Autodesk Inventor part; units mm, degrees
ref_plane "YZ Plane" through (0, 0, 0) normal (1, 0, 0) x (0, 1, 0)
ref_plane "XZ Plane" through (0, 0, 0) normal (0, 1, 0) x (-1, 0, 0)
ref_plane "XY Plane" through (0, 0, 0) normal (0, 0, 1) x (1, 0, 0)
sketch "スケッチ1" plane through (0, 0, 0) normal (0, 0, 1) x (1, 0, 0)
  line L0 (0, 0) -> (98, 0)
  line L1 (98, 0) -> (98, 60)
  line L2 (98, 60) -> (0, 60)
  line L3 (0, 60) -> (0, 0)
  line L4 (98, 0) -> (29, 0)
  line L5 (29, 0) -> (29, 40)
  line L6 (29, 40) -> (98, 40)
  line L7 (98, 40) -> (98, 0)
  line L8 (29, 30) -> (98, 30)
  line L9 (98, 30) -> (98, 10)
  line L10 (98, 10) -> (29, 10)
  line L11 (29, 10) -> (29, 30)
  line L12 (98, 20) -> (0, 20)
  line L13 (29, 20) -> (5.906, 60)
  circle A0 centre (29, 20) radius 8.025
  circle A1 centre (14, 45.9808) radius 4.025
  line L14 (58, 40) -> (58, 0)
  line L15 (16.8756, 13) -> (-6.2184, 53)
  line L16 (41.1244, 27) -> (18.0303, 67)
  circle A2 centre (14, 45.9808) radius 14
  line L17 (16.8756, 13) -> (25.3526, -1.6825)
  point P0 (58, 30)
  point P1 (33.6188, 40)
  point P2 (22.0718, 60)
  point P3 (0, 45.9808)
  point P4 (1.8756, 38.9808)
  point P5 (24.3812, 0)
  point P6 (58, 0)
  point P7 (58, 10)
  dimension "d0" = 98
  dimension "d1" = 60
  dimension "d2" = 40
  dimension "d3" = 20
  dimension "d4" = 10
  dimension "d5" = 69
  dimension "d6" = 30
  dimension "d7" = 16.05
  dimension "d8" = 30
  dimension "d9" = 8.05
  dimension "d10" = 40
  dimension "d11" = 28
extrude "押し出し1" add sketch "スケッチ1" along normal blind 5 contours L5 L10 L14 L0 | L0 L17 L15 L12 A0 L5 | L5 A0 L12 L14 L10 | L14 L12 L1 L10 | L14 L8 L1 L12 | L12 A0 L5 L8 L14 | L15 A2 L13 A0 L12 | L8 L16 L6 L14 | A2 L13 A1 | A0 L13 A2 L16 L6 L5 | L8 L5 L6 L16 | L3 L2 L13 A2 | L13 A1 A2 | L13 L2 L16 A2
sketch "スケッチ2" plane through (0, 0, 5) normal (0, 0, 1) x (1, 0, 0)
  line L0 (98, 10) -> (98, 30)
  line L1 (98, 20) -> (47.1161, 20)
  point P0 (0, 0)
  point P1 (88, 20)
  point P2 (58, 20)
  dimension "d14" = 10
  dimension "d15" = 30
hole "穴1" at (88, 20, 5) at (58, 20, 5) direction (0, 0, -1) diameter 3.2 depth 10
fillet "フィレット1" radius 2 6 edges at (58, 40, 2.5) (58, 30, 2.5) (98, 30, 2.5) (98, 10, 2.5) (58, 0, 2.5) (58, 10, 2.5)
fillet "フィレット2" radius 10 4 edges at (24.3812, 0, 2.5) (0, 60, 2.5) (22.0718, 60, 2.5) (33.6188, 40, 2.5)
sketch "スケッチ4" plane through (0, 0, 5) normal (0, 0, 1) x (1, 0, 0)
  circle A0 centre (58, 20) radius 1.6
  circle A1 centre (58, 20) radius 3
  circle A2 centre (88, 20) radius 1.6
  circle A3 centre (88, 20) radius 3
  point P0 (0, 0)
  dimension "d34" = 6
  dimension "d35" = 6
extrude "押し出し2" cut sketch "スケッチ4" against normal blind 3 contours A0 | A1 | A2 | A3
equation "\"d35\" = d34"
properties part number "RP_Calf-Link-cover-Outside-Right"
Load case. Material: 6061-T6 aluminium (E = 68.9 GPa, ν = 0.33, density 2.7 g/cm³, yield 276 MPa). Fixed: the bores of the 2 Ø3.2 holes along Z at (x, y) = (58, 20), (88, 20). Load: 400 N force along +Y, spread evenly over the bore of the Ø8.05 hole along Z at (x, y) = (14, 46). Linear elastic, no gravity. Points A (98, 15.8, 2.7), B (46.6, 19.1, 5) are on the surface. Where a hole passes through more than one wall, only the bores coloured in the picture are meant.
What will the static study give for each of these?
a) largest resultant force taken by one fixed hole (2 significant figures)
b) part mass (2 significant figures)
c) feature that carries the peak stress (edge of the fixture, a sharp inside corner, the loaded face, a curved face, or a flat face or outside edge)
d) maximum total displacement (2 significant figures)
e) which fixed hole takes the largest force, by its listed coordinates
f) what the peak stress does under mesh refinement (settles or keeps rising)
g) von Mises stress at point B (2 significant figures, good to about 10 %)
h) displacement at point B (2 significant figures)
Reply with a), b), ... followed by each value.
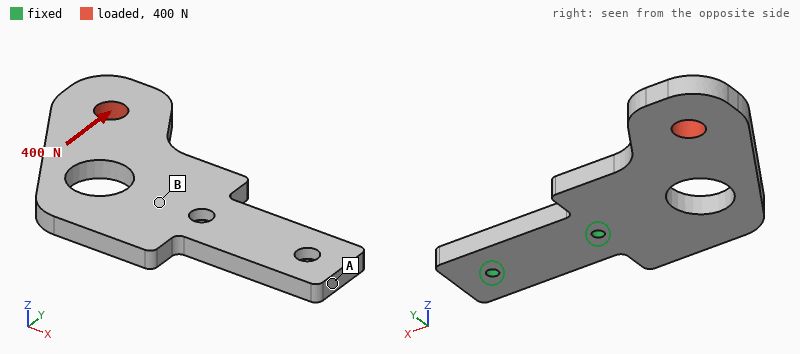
a) 930 N
b) 38 g
c) edge of the fixture
d) 0.13 mm
e) (58, 20)
f) keeps rising
g) 18 MPa
h) 0.023 mm
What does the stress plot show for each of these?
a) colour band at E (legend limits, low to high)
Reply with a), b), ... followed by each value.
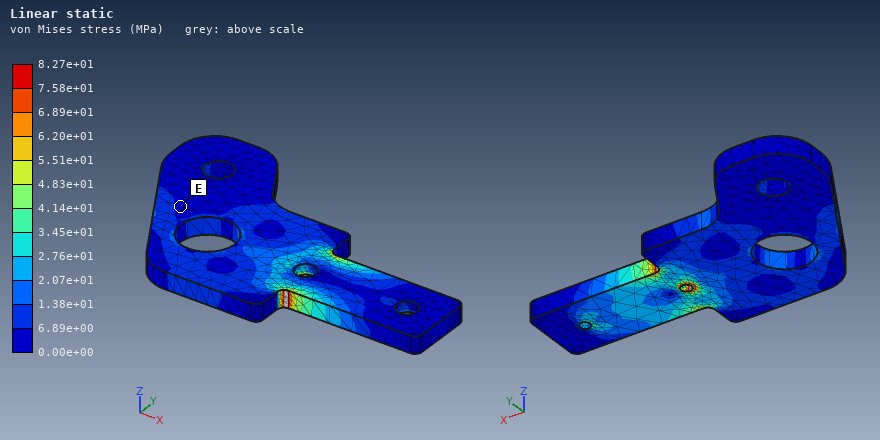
a) 0.00e+00 to 6.89e+00 MPa
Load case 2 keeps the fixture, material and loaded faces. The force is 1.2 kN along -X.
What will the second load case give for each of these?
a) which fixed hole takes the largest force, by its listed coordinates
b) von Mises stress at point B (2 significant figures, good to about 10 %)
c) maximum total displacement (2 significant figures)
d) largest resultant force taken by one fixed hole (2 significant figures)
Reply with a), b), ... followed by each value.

a) (58, 20)
b) 21 MPa
c) 0.22 mm
d) 1.3 kN
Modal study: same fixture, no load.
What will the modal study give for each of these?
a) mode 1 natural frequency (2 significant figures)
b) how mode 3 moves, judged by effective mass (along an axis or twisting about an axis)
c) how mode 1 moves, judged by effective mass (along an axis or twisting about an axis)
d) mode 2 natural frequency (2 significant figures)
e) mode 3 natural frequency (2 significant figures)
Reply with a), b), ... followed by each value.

a) 800 Hz
b) along Y
c) along Z
d) 2000 Hz
e) 2700 Hz
